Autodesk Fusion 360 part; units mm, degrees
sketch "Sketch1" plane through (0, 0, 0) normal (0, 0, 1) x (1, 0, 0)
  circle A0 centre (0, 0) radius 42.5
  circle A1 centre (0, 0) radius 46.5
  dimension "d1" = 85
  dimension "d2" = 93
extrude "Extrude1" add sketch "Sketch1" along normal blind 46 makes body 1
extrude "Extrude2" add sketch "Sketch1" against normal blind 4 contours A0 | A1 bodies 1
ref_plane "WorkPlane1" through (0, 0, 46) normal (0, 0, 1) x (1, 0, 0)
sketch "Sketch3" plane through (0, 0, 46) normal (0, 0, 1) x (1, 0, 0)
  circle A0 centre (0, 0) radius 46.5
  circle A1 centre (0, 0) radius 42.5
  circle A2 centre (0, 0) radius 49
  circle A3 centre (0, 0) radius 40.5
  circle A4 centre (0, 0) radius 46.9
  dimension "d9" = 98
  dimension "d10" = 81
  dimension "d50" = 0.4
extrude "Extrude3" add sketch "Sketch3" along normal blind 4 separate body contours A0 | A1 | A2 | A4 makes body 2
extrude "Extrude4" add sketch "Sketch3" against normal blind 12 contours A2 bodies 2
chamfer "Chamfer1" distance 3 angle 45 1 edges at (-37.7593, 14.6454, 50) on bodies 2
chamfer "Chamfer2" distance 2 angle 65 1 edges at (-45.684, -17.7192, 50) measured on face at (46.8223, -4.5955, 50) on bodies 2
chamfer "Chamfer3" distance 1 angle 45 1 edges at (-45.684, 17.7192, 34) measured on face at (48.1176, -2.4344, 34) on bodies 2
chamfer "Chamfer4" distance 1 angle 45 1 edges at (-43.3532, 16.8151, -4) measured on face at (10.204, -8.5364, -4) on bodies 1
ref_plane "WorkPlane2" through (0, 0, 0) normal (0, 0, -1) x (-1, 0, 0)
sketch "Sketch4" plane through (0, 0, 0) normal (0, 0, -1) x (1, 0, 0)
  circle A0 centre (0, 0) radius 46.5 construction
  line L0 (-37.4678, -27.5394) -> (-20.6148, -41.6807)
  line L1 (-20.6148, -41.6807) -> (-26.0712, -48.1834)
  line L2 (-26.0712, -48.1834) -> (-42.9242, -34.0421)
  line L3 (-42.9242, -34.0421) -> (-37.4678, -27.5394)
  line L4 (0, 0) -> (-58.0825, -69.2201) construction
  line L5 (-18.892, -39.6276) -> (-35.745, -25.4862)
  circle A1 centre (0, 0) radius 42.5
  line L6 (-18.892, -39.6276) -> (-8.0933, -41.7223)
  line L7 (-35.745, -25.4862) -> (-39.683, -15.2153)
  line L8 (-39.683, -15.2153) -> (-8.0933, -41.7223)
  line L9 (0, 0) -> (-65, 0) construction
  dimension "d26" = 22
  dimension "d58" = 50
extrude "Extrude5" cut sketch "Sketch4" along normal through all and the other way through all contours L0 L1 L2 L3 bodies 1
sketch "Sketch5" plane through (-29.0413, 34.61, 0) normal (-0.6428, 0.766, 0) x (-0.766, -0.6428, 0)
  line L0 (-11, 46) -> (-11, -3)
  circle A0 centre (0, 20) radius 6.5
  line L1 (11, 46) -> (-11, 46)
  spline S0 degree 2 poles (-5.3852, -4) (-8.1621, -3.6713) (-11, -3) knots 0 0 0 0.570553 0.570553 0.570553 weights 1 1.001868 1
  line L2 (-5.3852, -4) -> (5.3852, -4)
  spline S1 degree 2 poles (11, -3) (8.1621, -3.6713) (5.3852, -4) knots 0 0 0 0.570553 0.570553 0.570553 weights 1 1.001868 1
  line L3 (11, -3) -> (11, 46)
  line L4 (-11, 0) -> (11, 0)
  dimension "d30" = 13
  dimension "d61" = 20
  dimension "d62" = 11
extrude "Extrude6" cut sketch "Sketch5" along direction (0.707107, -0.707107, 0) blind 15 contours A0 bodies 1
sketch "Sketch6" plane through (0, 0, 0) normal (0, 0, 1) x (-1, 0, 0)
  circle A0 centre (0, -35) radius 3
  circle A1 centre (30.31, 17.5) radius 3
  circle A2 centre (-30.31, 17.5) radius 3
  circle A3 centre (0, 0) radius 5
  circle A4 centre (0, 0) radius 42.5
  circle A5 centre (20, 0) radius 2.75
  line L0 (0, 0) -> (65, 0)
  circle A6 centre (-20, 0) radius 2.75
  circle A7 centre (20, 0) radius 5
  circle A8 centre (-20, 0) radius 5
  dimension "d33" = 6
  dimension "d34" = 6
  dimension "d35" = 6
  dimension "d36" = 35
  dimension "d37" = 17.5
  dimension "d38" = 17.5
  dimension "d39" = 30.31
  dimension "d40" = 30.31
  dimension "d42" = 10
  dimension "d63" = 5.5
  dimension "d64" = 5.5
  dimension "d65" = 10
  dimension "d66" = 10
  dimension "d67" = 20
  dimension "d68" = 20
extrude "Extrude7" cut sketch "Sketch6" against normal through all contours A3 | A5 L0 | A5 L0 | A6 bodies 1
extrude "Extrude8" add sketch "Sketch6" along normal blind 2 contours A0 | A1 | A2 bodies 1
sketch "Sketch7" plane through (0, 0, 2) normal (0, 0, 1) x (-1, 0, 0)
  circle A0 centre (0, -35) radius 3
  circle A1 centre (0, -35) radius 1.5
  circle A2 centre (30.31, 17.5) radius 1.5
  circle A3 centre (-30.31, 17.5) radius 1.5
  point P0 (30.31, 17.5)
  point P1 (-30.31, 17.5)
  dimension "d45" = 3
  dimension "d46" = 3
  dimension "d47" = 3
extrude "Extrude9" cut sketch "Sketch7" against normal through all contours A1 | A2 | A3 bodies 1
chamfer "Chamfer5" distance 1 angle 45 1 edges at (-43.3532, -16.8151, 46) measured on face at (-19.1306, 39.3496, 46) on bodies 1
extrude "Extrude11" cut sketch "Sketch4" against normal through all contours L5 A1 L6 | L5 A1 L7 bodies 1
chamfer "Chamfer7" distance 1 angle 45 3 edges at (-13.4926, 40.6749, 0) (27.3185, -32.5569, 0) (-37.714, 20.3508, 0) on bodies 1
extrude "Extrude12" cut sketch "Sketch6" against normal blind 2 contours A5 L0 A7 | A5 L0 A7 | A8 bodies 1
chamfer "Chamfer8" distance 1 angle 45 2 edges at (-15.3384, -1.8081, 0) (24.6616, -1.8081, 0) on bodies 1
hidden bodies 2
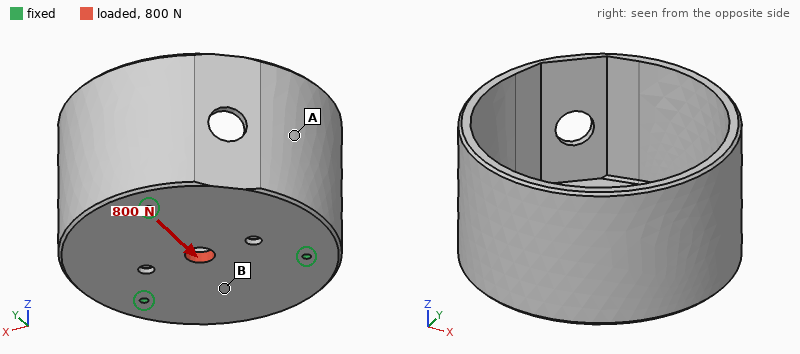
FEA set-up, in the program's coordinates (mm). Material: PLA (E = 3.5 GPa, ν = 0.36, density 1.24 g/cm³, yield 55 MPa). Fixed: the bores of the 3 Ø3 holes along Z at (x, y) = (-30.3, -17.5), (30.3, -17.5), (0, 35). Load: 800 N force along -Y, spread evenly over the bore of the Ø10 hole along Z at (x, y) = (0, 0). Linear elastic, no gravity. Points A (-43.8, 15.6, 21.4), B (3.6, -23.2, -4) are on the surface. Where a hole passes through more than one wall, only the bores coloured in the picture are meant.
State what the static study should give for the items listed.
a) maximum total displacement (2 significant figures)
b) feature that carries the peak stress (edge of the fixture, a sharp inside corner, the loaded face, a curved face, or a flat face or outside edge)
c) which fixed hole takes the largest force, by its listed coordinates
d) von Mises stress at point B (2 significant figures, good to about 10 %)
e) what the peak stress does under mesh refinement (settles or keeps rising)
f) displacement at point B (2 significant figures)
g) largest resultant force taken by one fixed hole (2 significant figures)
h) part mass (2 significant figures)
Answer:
51 µm
edge of the fixture
(0, 35)
1.8 MPa
keeps rising
32 µm
300 N
94 g
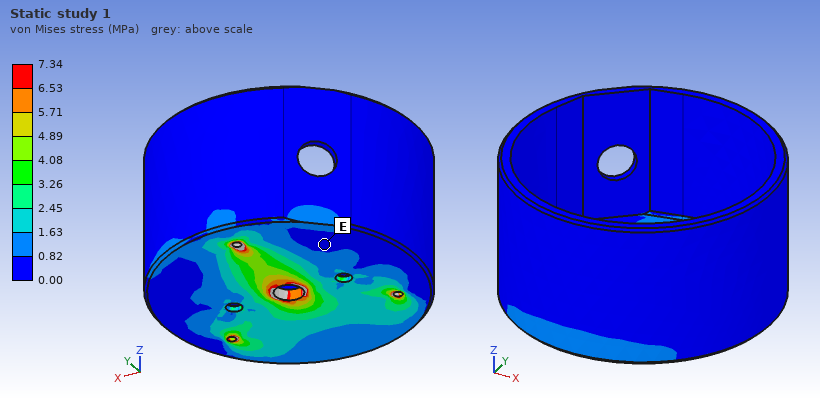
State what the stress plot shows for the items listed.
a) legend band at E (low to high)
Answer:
0.00 to 0.82 MPa
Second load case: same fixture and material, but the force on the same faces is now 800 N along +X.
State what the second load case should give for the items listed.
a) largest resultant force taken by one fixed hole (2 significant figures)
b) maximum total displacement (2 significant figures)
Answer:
280 N
53 µm
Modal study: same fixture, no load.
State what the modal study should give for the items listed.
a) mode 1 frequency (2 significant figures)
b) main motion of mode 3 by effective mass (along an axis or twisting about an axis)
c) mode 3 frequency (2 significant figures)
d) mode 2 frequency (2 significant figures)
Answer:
570 Hz
along X
1100 Hz
590 Hz
